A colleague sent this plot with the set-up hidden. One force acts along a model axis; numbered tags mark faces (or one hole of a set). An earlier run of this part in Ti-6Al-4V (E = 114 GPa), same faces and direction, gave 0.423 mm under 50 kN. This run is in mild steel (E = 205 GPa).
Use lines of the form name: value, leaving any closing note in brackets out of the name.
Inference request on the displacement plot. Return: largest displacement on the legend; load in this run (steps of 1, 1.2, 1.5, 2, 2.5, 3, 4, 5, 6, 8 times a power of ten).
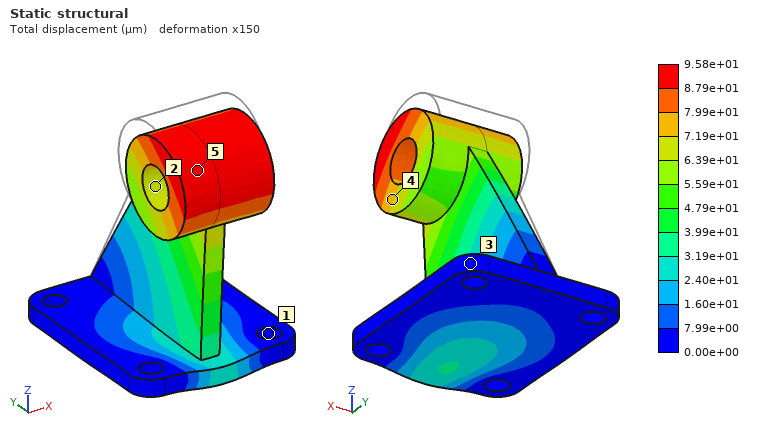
largest displacement on the legend: 9.58e+01 µm
load in this run: 20 kN
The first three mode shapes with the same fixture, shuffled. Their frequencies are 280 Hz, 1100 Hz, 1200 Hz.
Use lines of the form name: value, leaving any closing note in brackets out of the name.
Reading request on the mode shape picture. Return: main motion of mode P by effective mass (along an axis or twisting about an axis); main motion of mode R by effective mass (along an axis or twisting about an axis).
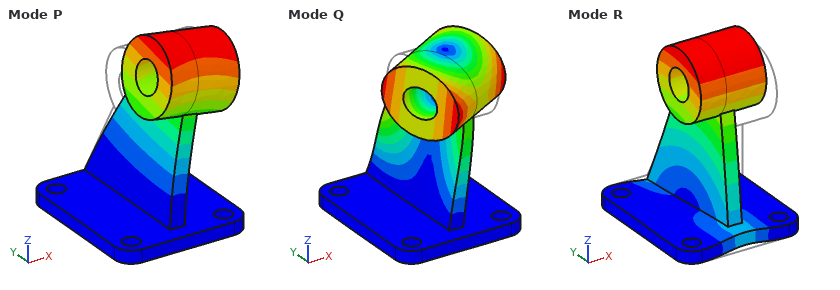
main motion of mode P by effective mass: along X
main motion of mode R by effective mass: along Y
